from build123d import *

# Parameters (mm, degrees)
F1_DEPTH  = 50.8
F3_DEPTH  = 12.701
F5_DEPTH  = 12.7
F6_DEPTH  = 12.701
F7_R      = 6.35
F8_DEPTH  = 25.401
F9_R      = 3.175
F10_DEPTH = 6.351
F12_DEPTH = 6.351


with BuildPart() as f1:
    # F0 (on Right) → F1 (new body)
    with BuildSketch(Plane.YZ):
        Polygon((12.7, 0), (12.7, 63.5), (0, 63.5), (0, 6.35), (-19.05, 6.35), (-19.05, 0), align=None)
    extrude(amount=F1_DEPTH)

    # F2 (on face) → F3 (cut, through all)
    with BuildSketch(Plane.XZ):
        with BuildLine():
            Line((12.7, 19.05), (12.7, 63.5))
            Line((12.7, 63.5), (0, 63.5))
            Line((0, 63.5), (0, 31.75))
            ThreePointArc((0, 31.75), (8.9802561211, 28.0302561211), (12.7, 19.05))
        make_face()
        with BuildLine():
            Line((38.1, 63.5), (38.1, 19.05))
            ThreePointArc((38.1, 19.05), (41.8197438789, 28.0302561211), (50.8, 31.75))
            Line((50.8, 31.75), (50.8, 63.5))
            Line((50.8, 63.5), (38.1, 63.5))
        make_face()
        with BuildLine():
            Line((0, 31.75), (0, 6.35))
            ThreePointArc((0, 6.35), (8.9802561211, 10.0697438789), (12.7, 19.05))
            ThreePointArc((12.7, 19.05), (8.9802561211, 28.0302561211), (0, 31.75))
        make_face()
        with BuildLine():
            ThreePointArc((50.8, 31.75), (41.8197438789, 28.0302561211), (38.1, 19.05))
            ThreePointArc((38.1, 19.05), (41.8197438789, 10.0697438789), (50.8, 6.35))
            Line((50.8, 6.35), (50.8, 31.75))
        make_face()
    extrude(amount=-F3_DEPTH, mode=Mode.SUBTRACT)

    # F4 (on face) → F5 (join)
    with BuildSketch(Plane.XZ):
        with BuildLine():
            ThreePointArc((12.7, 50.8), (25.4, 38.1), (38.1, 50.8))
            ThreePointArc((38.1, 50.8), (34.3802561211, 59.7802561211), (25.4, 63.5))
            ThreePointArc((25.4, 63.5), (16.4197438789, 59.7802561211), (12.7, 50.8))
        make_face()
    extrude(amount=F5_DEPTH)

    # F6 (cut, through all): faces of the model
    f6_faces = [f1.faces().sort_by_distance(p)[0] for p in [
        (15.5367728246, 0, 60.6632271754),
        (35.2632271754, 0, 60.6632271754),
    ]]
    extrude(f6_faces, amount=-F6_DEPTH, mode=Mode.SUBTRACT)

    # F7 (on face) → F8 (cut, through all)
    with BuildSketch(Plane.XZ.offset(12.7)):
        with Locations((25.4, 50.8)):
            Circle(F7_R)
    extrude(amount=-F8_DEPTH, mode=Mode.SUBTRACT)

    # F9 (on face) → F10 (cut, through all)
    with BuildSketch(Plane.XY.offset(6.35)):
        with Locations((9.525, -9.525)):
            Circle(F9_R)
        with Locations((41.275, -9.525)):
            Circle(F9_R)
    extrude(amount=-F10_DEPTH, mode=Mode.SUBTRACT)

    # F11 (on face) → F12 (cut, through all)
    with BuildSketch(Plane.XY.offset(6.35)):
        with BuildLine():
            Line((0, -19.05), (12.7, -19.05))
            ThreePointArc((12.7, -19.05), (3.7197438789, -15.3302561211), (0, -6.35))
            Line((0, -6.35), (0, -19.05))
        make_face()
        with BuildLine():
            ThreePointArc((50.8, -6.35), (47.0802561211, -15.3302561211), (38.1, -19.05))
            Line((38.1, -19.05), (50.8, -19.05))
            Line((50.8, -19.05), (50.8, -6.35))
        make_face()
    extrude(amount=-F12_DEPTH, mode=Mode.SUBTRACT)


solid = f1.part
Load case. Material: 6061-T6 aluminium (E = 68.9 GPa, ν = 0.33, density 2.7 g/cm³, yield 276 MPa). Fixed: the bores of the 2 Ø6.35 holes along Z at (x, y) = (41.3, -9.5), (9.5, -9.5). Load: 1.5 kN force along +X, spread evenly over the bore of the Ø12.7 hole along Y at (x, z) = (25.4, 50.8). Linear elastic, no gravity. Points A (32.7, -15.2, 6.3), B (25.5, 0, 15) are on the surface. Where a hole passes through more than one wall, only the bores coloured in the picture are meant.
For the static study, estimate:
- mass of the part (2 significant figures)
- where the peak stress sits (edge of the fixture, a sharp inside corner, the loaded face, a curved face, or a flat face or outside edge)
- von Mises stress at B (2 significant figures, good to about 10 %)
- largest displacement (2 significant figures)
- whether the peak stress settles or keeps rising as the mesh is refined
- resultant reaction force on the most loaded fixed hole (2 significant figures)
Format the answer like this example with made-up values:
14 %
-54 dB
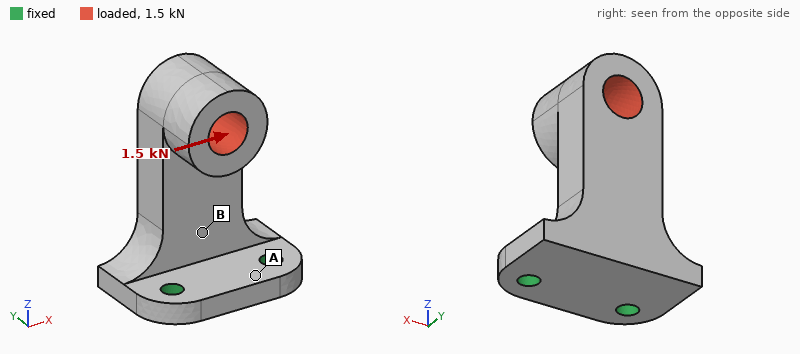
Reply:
84 g
edge of the fixture
29 MPa
0.19 mm
keeps rising
2.3 kN
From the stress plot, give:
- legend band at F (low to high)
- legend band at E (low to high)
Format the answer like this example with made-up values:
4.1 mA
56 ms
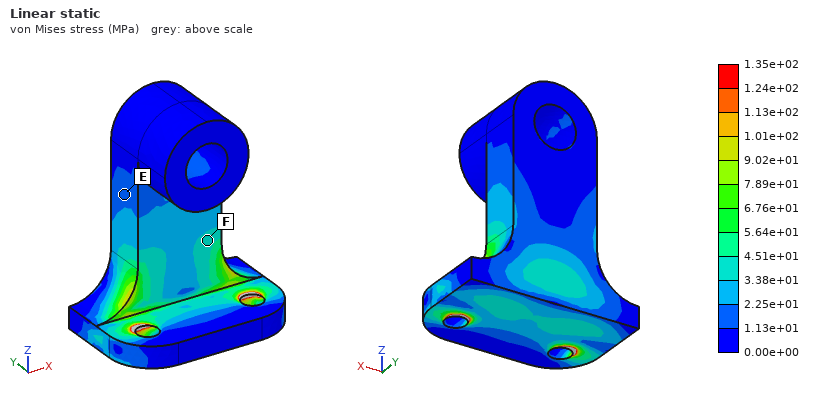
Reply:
3.38e+01 to 4.51e+01 MPa
1.13e+01 to 2.25e+01 MPa
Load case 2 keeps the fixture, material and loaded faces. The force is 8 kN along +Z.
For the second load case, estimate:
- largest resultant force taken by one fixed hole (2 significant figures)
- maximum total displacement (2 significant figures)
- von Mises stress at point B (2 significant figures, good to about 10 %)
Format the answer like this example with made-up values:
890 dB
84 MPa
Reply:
4.0 kN
0.15 mm
71 MPa
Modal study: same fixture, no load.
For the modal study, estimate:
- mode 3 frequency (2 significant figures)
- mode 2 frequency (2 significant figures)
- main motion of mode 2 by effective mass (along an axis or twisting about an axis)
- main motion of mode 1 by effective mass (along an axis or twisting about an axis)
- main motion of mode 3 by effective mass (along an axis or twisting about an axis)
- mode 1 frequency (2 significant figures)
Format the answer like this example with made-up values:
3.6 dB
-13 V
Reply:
5900 Hz
2900 Hz
along X
along Y
along Z
1200 Hz
